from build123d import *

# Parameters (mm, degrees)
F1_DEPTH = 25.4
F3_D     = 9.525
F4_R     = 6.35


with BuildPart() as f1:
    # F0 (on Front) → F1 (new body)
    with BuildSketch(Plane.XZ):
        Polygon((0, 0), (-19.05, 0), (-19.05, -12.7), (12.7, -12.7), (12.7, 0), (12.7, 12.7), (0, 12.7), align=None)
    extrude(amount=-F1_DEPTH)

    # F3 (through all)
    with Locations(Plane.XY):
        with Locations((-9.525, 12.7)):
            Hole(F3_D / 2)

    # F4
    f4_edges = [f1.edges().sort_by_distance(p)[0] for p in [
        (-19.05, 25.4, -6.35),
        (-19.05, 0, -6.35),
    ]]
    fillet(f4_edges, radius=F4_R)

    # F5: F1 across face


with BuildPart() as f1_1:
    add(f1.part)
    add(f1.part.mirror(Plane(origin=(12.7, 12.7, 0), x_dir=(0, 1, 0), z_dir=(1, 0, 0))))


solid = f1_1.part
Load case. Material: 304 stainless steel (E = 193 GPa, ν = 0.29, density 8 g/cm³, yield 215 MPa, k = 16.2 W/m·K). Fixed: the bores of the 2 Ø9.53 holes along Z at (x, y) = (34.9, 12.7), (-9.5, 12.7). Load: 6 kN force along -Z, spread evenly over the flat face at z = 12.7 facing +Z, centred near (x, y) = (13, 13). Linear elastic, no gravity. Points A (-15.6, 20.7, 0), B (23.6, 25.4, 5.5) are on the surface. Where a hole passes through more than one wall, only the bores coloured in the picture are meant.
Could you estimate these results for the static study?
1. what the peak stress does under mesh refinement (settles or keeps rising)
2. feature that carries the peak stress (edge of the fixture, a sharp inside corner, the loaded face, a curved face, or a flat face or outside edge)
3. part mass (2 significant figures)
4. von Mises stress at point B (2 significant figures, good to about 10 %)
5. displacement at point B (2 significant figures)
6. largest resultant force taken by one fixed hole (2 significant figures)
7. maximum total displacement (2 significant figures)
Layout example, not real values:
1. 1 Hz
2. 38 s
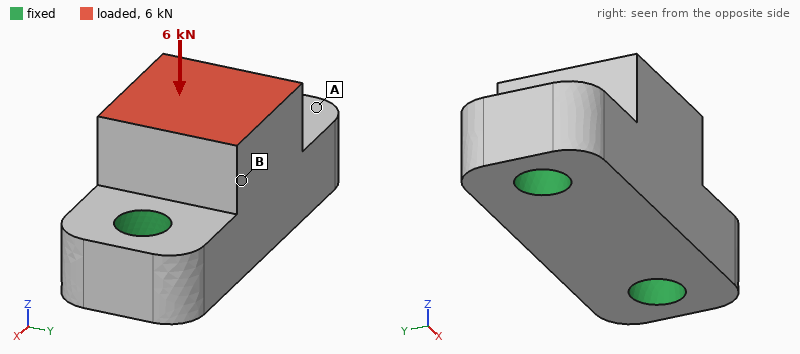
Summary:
1. keeps rising
2. edge of the fixture
3. 210 g
4. 11 MPa
5. 2.5 µm
6. 3.1 kN
7. 2.9 µm
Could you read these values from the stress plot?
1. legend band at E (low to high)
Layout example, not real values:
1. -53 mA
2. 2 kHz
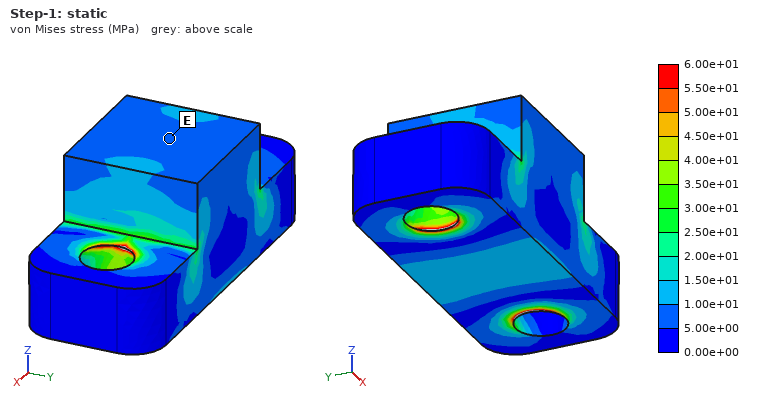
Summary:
1. 5.00e+00 to 1.00e+01 MPa
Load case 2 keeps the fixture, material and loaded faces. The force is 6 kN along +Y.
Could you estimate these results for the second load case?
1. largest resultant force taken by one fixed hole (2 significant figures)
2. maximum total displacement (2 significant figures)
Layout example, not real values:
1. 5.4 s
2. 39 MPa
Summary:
1. 3.0 kN
2. 19 µm
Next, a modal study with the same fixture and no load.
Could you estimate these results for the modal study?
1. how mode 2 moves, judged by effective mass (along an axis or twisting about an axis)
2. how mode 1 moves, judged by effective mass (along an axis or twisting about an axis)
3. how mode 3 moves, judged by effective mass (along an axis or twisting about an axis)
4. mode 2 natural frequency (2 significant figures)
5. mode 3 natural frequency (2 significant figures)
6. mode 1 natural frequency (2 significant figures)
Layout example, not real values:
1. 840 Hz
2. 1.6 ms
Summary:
1. along Z
2. along Y
3. along X
4. 22 kHz
5. 27 kHz
6. 14 kHz
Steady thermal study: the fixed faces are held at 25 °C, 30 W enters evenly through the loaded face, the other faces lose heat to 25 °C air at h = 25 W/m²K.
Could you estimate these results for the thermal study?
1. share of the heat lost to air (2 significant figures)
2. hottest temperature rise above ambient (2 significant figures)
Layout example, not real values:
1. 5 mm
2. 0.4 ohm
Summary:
1. 10 %
2. 74 K
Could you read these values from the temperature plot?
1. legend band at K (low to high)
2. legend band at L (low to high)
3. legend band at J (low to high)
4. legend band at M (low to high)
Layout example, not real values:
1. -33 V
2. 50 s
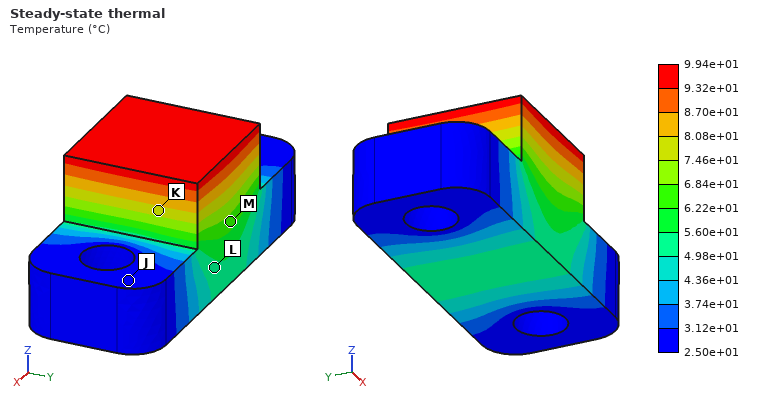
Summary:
1. 7.46e+01 to 8.08e+01 °C
2. 4.98e+01 to 5.60e+01 °C
3. 2.50e+01 to 3.12e+01 °C
4. 6.22e+01 to 6.84e+01 °C
